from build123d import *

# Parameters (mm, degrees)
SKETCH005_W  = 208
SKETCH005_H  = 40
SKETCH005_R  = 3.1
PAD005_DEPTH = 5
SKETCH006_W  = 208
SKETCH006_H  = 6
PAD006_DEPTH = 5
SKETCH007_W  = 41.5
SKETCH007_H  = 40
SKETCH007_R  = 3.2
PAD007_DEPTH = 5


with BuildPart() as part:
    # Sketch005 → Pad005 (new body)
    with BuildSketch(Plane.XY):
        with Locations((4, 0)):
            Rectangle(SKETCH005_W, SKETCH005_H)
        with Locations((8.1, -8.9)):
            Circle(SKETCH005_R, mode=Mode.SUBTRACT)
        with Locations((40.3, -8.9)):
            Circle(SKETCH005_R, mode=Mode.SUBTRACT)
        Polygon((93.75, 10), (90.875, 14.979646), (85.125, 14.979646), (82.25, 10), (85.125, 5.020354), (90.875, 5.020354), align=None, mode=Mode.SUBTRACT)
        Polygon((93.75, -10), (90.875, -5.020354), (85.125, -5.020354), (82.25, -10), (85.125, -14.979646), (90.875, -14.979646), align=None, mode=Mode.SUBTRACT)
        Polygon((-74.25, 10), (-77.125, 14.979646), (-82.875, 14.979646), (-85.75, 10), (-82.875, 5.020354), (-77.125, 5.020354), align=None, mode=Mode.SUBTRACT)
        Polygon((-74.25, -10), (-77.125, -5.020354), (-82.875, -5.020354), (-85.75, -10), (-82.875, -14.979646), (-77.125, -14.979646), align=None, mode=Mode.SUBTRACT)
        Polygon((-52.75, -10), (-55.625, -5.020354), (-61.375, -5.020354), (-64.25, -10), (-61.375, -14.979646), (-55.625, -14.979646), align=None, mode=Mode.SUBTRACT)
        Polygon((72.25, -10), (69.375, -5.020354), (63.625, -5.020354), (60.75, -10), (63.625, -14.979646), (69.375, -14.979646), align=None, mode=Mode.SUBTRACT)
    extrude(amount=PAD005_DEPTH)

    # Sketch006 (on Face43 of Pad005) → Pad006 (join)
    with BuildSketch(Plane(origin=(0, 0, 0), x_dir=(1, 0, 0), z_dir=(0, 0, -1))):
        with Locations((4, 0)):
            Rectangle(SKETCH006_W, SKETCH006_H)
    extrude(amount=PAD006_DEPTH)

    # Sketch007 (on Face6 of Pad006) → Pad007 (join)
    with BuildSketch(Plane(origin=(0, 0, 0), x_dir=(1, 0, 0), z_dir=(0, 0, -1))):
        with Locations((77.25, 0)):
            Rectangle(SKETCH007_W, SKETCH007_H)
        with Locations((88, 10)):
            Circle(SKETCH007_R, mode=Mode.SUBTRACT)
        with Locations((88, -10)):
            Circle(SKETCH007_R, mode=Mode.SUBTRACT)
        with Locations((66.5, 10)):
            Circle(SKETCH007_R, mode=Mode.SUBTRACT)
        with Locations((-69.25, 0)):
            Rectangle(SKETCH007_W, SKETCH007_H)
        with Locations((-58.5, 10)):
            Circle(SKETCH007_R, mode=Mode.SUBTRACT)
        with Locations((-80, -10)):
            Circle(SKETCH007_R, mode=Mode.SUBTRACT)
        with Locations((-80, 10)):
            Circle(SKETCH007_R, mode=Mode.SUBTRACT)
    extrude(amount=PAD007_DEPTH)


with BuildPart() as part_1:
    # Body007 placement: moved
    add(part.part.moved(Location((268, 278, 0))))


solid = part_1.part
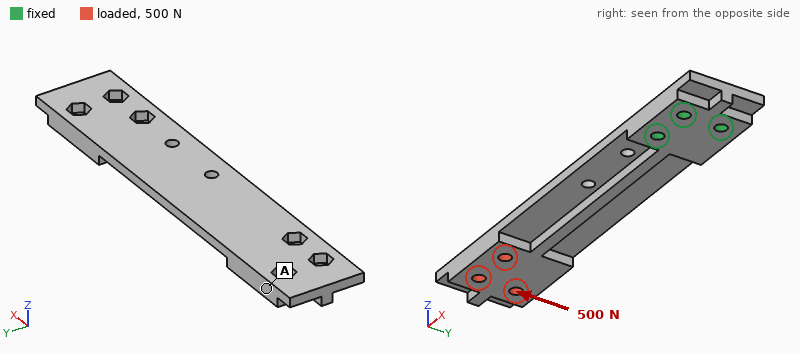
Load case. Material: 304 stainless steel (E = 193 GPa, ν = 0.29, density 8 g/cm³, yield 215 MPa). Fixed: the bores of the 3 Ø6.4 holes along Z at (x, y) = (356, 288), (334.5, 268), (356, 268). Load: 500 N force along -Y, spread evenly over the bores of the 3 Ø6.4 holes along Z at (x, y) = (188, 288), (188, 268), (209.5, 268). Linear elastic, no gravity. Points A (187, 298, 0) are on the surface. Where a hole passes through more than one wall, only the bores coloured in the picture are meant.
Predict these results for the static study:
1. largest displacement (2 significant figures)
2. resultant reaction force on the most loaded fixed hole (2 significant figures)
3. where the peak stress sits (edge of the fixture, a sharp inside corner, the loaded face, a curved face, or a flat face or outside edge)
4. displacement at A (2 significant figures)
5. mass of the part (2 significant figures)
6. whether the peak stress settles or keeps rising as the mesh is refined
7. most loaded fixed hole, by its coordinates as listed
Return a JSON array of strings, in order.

["0.16 mm", "2.2 kN", "edge of the fixture", "0.13 mm", "460 g", "keeps rising", "(334.5, 268)"]
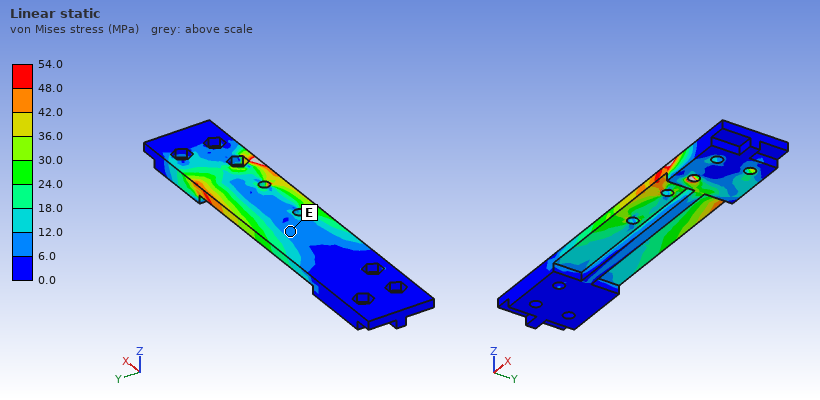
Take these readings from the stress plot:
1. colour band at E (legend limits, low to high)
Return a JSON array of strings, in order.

["6.0 to 12.0 MPa"]
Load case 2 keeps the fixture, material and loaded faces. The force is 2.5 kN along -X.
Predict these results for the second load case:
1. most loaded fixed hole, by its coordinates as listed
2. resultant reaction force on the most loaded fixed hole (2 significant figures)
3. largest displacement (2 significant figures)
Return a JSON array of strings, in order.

["(334.5, 268)", "1.5 kN", "0.61 mm"]
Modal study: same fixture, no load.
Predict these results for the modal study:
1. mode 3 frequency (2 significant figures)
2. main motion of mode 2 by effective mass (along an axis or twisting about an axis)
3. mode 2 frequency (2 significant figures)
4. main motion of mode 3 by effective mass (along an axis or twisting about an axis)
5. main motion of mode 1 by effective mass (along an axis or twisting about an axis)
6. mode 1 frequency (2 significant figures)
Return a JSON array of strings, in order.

["1200 Hz", "along Y", "810 Hz", "twisting about X", "along Z", "190 Hz"]
